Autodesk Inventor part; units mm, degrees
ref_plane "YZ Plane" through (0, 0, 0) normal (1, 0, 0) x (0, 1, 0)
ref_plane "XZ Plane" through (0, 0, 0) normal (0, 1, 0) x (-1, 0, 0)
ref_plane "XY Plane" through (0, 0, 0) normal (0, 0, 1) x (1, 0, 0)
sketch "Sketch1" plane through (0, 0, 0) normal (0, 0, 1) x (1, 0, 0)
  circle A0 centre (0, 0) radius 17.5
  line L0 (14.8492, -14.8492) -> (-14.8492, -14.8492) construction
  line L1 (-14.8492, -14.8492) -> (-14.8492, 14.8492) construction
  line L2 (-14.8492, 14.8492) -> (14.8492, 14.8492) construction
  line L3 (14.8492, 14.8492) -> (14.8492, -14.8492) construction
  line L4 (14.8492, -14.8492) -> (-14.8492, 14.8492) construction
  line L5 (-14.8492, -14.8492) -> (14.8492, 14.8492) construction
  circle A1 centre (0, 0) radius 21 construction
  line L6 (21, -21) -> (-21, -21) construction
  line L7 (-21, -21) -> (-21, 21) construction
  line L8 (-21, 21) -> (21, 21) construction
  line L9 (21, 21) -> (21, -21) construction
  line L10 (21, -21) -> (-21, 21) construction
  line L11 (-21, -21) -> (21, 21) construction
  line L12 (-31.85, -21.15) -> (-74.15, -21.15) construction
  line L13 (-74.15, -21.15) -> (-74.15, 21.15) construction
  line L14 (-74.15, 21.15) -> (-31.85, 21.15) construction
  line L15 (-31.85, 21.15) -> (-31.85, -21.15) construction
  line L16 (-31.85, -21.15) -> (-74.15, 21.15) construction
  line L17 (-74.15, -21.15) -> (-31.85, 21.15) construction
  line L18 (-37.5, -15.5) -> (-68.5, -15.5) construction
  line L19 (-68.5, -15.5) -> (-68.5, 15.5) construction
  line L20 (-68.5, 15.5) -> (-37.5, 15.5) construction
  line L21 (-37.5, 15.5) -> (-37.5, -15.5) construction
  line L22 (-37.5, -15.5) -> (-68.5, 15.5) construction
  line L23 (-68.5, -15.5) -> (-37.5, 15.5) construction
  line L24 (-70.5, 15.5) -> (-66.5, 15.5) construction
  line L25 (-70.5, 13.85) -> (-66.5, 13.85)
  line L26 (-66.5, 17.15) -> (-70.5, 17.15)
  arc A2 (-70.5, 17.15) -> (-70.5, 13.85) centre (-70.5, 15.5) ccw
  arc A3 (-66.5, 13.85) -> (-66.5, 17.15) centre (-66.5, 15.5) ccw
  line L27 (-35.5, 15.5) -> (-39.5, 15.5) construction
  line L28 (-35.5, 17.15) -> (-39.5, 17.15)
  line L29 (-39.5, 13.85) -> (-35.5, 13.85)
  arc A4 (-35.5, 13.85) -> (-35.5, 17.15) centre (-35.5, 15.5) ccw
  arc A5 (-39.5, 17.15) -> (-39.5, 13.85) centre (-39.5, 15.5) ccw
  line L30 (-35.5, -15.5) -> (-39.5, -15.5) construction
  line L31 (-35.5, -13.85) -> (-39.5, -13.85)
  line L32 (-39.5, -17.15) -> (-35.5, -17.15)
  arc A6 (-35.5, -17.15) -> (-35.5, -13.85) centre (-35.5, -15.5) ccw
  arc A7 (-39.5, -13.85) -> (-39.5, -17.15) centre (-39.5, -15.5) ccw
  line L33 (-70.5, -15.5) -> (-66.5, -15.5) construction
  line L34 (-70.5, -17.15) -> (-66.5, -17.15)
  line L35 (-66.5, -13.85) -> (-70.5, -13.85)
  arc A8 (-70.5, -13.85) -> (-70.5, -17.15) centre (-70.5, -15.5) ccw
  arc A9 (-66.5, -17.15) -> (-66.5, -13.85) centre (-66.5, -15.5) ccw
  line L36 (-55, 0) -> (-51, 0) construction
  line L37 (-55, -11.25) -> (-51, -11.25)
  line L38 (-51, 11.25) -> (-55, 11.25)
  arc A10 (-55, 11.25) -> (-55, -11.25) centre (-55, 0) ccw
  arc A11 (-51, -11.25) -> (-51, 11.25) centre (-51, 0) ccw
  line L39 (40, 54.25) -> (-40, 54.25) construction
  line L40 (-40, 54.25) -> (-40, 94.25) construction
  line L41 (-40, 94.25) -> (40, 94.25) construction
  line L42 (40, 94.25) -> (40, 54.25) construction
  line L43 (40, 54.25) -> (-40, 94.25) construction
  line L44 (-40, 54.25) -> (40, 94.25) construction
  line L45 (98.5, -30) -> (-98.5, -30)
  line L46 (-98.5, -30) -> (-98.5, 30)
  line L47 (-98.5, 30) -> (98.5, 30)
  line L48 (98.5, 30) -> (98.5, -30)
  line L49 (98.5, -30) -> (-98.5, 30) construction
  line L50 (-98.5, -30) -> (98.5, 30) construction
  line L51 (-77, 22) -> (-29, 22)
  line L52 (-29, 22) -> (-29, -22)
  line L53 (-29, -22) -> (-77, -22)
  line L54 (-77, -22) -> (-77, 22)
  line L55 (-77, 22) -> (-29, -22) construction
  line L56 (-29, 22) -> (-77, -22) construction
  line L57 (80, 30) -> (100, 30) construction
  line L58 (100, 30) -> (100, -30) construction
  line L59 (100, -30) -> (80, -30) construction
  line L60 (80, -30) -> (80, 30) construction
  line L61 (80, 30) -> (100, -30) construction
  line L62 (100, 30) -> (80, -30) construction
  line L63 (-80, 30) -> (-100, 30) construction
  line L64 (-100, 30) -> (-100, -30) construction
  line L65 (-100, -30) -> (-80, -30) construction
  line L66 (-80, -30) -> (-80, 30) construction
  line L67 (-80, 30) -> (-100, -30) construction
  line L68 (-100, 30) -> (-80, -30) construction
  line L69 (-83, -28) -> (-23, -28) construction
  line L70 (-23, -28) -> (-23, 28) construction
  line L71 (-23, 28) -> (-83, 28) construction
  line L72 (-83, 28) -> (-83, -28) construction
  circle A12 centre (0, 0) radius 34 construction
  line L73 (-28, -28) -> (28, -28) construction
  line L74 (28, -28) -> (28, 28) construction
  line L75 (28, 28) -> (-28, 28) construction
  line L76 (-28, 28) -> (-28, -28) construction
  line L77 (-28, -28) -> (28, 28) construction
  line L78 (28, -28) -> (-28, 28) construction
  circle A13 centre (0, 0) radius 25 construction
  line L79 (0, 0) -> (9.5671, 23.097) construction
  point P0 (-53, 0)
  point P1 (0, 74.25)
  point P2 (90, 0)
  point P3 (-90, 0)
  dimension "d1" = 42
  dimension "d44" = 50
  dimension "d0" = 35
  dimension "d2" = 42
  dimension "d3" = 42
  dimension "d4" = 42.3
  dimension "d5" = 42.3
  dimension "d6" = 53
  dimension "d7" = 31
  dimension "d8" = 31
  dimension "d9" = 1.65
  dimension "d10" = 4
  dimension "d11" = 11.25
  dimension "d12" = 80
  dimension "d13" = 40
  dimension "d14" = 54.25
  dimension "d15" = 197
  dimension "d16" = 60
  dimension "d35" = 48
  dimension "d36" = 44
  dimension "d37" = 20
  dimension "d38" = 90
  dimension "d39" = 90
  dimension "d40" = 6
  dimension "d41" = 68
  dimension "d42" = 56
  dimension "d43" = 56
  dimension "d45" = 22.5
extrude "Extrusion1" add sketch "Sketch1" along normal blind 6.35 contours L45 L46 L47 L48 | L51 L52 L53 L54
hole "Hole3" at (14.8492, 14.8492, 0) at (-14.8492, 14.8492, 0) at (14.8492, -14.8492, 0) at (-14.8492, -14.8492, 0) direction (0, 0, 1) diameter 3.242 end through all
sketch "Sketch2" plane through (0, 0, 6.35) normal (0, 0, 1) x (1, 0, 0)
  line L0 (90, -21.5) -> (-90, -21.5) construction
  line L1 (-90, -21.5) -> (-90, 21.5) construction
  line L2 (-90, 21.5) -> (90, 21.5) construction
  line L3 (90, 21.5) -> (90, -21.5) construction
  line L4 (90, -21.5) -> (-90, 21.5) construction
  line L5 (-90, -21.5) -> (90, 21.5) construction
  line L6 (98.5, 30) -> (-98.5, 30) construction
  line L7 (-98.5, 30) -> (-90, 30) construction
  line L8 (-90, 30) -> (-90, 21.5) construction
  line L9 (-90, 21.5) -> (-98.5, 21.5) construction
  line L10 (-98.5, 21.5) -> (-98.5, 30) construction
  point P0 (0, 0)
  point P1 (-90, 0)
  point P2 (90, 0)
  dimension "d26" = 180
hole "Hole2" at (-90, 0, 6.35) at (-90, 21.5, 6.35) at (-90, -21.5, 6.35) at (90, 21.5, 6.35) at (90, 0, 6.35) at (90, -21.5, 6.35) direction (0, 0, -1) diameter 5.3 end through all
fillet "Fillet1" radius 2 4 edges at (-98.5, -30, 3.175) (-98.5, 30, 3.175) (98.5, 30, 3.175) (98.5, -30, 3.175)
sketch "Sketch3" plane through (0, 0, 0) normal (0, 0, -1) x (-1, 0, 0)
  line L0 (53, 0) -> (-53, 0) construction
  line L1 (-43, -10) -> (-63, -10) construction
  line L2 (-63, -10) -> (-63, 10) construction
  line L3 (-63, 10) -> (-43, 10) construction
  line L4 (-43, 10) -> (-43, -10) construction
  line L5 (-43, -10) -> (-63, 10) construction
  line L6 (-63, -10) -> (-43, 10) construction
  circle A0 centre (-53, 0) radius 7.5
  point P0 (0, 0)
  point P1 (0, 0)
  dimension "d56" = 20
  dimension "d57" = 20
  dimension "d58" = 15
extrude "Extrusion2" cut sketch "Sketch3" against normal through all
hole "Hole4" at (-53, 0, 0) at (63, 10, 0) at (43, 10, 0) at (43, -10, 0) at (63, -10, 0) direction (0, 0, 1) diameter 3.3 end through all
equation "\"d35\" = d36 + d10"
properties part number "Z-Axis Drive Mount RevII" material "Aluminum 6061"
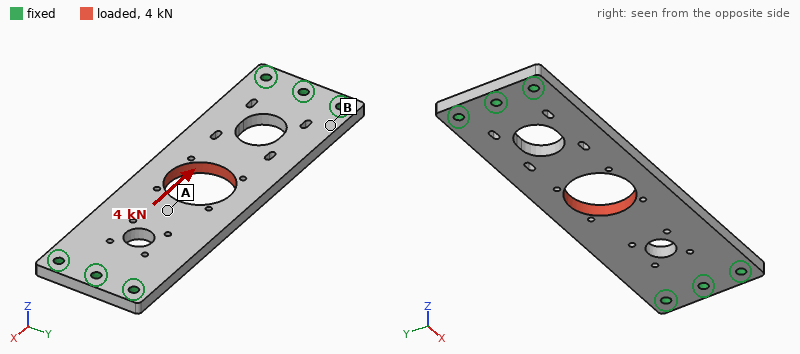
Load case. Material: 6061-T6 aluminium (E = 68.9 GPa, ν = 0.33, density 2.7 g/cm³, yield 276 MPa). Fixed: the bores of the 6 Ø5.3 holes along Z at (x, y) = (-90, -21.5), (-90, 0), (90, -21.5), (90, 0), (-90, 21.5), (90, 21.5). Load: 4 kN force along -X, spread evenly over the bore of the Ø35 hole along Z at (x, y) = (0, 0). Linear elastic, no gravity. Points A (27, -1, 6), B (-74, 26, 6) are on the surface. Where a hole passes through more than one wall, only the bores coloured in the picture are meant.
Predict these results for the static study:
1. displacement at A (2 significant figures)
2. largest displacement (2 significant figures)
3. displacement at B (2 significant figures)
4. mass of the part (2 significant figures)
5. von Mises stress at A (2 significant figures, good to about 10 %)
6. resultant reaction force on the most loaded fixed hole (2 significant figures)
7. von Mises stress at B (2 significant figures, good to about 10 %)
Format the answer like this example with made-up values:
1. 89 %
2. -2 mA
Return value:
1. 6.6 µm
2. 9.2 µm
3. 2.2 µm
4. 170 g
5. 5.3 MPa
6. 760 N
7. 8.1 MPa
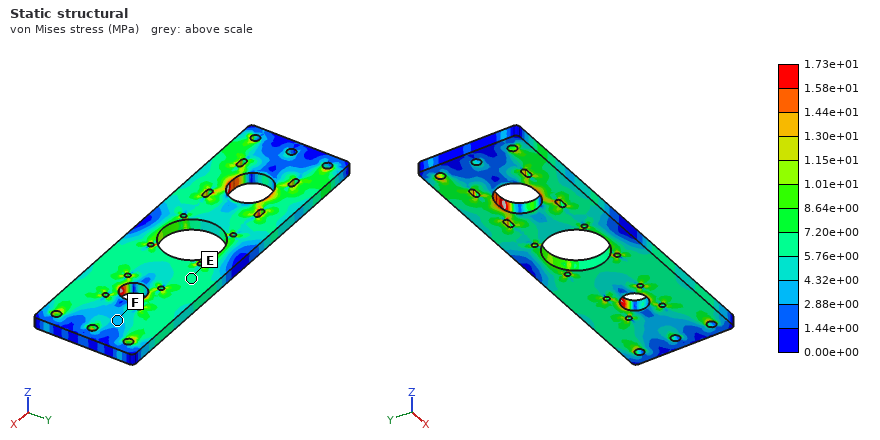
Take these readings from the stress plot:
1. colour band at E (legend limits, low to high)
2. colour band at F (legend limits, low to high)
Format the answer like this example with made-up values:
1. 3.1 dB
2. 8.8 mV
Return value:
1. 5.76e+00 to 7.20e+00 MPa
2. 2.88e+00 to 4.32e+00 MPa
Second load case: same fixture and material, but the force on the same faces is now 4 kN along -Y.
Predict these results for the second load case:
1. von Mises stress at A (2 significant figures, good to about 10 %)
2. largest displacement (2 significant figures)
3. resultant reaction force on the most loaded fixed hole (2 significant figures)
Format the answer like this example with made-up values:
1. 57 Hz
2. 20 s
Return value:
1. 18 MPa
2. 50 µm
3. 2.2 kN
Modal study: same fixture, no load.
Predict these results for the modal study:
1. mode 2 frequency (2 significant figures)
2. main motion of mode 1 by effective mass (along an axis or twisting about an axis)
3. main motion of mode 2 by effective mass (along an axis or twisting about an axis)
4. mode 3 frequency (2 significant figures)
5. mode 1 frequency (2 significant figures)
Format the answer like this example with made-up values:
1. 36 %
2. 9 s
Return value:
1. 2000 Hz
2. along Z
3. twisting about X
4. 2700 Hz
5. 1000 Hz
